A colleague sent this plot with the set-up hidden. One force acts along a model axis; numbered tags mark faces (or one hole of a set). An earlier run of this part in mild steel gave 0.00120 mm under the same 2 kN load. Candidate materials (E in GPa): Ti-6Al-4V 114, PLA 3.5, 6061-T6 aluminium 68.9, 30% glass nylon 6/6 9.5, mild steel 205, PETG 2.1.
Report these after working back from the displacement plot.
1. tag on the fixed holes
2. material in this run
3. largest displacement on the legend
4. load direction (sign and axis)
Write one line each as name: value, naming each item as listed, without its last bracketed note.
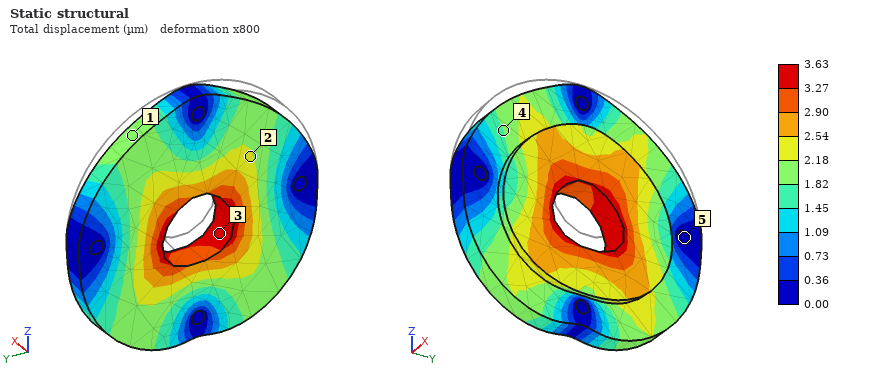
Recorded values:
tag on the fixed holes: 5
material in this run: 6061-T6 aluminium
largest displacement on the legend: 3.63 µm
load direction: -Z
